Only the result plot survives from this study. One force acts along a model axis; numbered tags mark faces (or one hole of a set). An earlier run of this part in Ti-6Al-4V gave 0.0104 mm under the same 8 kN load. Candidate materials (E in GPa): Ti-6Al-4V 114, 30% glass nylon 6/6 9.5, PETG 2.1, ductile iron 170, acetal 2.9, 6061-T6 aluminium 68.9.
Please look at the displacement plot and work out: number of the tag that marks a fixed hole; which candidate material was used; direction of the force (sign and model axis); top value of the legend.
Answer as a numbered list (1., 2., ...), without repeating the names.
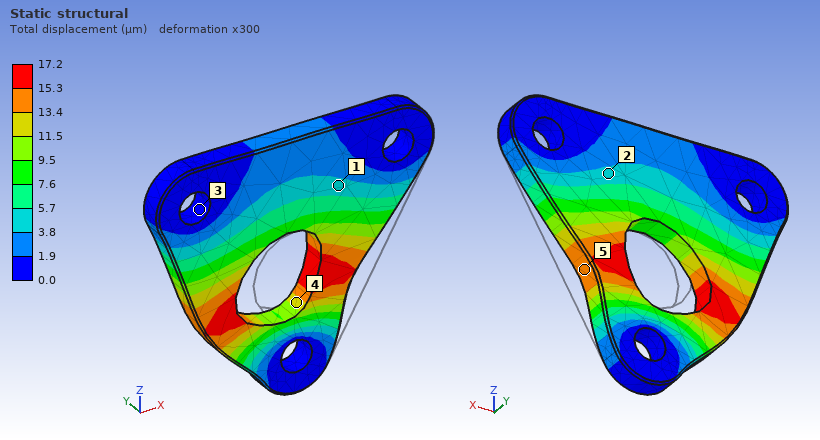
1. 3
2. 6061-T6 aluminium
3. -X
4. 17.2 µm
